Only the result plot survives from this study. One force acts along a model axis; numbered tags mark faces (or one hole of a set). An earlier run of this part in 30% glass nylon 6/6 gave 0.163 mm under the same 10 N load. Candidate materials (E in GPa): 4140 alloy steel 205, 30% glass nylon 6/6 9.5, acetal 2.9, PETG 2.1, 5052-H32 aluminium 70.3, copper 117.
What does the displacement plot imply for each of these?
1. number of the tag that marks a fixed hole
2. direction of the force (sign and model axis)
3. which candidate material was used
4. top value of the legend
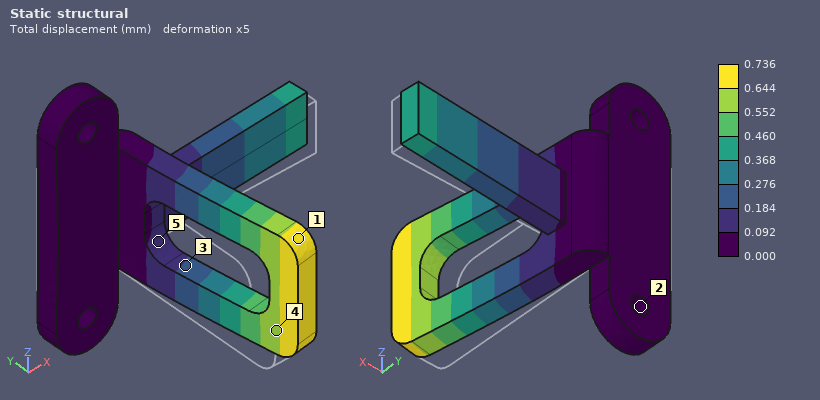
2
+X
PETG
0.736 mm
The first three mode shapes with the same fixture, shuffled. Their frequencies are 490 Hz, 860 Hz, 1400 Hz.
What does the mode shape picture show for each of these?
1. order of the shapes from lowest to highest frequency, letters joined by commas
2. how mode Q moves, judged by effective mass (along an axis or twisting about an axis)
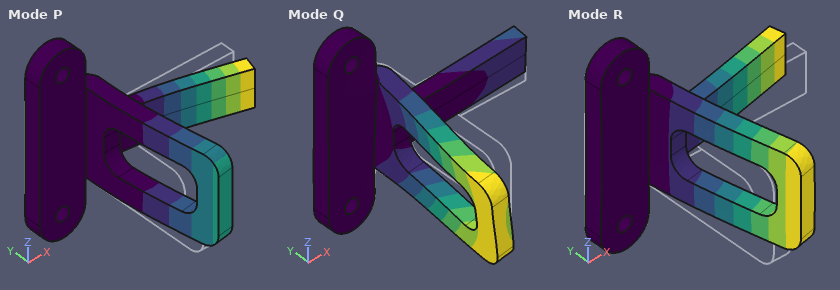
R, P, Q
along Z
